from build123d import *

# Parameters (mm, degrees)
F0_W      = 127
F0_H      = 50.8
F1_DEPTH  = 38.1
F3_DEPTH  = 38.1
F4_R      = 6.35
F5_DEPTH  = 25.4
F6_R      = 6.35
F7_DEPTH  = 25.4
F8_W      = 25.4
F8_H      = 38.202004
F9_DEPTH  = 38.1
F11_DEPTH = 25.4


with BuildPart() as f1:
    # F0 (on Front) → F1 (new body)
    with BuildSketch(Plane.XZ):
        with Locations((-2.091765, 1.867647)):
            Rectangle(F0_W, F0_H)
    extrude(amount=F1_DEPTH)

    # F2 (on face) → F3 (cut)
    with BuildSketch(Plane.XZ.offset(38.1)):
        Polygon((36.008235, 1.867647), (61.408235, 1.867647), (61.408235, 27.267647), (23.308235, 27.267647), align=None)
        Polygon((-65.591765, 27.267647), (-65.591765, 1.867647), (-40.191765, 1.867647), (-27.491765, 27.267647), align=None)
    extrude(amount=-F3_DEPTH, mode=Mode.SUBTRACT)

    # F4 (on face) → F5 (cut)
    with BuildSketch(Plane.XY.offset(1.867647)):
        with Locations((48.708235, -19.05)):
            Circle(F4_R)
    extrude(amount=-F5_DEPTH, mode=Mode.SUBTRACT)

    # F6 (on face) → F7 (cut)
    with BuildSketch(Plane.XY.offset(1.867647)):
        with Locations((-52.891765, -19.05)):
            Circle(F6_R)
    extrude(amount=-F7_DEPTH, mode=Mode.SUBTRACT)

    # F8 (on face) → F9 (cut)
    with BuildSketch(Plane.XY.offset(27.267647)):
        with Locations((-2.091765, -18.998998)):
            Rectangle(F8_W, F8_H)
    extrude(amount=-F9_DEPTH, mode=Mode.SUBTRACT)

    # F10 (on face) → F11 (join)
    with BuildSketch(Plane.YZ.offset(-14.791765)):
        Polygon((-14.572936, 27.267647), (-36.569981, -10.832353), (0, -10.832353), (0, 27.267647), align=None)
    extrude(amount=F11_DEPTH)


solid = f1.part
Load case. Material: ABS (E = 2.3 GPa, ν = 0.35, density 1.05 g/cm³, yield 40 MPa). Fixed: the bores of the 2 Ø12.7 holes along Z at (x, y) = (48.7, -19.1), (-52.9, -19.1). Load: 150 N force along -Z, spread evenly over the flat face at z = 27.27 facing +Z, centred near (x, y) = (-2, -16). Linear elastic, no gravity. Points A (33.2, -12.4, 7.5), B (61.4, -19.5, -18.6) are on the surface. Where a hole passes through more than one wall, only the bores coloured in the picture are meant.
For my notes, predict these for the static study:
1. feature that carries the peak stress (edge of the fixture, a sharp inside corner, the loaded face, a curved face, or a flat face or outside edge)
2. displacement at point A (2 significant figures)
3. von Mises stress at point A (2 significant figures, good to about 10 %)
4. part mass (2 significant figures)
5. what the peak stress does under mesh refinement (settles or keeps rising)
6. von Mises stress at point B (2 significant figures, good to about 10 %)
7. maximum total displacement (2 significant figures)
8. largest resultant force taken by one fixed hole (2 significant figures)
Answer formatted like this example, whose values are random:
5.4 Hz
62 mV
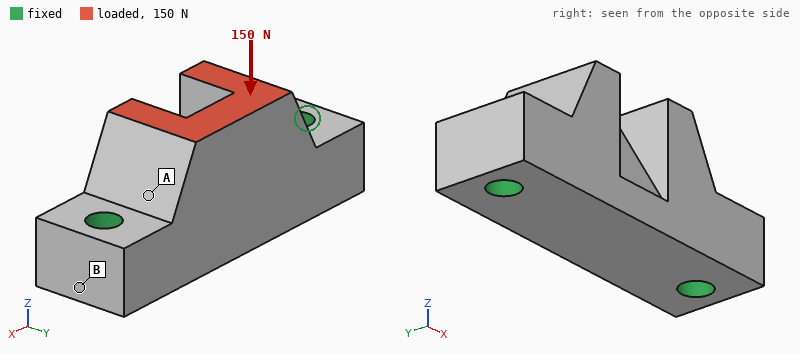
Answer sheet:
edge of the fixture
2.9 µm
0.19 MPa
170 g
keeps rising
0.061 MPa
7.6 µm
80 N
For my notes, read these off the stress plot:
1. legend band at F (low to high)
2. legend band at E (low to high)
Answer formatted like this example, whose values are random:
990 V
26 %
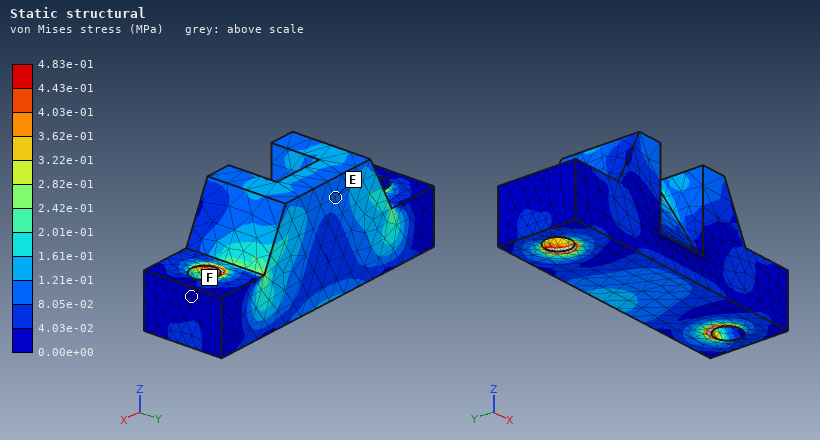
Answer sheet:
0.00e+00 to 4.03e-02 MPa
8.05e-02 to 1.21e-01 MPa
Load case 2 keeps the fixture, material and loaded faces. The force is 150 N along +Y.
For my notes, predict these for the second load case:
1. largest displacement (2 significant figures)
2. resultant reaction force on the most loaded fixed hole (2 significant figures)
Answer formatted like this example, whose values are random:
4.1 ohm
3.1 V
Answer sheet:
36 µm
75 N
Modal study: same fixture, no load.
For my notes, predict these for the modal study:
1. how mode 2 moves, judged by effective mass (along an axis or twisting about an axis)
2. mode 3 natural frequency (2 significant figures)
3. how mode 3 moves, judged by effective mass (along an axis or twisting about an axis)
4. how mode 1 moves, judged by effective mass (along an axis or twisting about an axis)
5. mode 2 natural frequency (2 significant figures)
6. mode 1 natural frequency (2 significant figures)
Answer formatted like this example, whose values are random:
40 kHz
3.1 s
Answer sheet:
along Z
3100 Hz
along Y
along Y
2800 Hz
1900 Hz
